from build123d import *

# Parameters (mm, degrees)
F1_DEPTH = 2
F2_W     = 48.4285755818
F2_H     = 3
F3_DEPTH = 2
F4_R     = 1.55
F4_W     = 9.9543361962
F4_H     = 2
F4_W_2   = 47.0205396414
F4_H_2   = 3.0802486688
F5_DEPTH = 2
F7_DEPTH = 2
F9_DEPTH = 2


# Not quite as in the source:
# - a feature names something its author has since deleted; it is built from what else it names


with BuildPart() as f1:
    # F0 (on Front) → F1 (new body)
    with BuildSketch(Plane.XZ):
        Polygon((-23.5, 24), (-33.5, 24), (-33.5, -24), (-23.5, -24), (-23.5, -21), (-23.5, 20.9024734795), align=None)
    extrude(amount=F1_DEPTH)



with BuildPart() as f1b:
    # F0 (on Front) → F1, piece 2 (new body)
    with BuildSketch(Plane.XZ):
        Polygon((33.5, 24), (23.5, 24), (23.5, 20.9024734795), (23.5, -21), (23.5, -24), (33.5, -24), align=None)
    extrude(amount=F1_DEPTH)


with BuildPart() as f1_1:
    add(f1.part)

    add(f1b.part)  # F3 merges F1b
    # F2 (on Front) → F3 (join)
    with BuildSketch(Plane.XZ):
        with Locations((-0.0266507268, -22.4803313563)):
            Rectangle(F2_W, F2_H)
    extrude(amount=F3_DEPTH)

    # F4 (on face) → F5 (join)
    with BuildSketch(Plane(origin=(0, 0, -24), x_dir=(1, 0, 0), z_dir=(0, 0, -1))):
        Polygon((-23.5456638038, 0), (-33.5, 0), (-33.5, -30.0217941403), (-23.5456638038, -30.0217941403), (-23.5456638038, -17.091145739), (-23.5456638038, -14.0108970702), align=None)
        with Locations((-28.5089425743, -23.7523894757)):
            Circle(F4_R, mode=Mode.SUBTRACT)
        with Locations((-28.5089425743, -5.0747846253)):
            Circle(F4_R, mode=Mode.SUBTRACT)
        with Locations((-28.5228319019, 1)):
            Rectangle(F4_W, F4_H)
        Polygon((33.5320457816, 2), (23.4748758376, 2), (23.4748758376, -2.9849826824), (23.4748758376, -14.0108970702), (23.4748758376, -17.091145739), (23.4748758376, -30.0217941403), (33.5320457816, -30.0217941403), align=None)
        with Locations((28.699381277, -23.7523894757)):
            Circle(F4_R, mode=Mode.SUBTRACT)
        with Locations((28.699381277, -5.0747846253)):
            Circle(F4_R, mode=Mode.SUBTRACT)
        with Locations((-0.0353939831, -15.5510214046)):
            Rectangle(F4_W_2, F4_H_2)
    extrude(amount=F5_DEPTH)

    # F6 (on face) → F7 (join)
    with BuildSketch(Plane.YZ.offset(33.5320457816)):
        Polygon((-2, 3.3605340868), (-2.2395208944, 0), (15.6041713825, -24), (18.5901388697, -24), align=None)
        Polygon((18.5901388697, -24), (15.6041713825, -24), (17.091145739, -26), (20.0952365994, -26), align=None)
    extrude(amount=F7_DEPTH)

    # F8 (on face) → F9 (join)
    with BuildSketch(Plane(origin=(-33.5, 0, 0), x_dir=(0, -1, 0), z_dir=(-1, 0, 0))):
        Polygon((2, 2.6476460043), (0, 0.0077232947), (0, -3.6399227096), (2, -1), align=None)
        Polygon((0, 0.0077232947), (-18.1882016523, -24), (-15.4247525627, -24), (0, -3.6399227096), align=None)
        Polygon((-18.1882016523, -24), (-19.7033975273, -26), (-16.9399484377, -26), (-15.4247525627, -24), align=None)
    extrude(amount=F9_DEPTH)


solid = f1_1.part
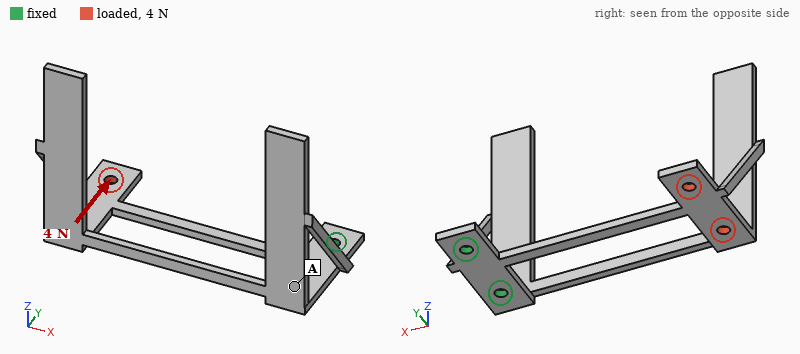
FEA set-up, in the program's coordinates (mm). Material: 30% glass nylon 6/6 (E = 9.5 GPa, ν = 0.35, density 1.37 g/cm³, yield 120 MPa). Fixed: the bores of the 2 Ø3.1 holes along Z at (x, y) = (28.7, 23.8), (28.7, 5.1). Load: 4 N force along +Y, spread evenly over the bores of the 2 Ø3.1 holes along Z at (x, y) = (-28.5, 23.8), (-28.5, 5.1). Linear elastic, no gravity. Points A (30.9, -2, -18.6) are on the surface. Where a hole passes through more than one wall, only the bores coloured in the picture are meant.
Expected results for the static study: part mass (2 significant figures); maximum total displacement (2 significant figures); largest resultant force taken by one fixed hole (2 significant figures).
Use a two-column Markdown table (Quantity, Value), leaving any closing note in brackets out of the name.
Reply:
| Quantity | Value |
|---|---|
| part mass | 5.5 g |
| maximum total displacement | 1.0 mm |
| largest resultant force taken by one fixed hole | 11 N |
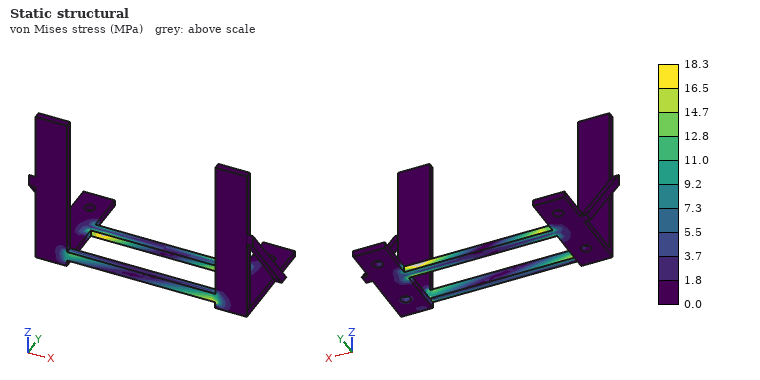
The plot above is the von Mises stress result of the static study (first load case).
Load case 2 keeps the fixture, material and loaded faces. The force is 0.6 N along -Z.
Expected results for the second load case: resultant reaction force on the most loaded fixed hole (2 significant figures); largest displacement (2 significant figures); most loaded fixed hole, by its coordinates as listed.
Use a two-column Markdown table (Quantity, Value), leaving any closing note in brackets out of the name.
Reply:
| Quantity | Value |
|---|---|
| resultant reaction force on the most loaded fixed hole | 0.38 N |
| largest displacement | 0.89 mm |
| most loaded fixed hole, by its coordinates as listed | (28.7, 23.8) |
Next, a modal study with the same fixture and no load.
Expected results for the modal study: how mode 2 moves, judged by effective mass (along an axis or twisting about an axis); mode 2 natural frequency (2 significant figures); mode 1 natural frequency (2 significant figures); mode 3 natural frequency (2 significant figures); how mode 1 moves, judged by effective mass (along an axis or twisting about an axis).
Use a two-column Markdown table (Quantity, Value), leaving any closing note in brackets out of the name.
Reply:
| Quantity | Value |
|---|---|
| how mode 2 moves, judged by effective mass | along Y |
| mode 2 natural frequency | 130 Hz |
| mode 1 natural frequency | 92 Hz |
| mode 3 natural frequency | 310 Hz |
| how mode 1 moves, judged by effective mass | along Z |
